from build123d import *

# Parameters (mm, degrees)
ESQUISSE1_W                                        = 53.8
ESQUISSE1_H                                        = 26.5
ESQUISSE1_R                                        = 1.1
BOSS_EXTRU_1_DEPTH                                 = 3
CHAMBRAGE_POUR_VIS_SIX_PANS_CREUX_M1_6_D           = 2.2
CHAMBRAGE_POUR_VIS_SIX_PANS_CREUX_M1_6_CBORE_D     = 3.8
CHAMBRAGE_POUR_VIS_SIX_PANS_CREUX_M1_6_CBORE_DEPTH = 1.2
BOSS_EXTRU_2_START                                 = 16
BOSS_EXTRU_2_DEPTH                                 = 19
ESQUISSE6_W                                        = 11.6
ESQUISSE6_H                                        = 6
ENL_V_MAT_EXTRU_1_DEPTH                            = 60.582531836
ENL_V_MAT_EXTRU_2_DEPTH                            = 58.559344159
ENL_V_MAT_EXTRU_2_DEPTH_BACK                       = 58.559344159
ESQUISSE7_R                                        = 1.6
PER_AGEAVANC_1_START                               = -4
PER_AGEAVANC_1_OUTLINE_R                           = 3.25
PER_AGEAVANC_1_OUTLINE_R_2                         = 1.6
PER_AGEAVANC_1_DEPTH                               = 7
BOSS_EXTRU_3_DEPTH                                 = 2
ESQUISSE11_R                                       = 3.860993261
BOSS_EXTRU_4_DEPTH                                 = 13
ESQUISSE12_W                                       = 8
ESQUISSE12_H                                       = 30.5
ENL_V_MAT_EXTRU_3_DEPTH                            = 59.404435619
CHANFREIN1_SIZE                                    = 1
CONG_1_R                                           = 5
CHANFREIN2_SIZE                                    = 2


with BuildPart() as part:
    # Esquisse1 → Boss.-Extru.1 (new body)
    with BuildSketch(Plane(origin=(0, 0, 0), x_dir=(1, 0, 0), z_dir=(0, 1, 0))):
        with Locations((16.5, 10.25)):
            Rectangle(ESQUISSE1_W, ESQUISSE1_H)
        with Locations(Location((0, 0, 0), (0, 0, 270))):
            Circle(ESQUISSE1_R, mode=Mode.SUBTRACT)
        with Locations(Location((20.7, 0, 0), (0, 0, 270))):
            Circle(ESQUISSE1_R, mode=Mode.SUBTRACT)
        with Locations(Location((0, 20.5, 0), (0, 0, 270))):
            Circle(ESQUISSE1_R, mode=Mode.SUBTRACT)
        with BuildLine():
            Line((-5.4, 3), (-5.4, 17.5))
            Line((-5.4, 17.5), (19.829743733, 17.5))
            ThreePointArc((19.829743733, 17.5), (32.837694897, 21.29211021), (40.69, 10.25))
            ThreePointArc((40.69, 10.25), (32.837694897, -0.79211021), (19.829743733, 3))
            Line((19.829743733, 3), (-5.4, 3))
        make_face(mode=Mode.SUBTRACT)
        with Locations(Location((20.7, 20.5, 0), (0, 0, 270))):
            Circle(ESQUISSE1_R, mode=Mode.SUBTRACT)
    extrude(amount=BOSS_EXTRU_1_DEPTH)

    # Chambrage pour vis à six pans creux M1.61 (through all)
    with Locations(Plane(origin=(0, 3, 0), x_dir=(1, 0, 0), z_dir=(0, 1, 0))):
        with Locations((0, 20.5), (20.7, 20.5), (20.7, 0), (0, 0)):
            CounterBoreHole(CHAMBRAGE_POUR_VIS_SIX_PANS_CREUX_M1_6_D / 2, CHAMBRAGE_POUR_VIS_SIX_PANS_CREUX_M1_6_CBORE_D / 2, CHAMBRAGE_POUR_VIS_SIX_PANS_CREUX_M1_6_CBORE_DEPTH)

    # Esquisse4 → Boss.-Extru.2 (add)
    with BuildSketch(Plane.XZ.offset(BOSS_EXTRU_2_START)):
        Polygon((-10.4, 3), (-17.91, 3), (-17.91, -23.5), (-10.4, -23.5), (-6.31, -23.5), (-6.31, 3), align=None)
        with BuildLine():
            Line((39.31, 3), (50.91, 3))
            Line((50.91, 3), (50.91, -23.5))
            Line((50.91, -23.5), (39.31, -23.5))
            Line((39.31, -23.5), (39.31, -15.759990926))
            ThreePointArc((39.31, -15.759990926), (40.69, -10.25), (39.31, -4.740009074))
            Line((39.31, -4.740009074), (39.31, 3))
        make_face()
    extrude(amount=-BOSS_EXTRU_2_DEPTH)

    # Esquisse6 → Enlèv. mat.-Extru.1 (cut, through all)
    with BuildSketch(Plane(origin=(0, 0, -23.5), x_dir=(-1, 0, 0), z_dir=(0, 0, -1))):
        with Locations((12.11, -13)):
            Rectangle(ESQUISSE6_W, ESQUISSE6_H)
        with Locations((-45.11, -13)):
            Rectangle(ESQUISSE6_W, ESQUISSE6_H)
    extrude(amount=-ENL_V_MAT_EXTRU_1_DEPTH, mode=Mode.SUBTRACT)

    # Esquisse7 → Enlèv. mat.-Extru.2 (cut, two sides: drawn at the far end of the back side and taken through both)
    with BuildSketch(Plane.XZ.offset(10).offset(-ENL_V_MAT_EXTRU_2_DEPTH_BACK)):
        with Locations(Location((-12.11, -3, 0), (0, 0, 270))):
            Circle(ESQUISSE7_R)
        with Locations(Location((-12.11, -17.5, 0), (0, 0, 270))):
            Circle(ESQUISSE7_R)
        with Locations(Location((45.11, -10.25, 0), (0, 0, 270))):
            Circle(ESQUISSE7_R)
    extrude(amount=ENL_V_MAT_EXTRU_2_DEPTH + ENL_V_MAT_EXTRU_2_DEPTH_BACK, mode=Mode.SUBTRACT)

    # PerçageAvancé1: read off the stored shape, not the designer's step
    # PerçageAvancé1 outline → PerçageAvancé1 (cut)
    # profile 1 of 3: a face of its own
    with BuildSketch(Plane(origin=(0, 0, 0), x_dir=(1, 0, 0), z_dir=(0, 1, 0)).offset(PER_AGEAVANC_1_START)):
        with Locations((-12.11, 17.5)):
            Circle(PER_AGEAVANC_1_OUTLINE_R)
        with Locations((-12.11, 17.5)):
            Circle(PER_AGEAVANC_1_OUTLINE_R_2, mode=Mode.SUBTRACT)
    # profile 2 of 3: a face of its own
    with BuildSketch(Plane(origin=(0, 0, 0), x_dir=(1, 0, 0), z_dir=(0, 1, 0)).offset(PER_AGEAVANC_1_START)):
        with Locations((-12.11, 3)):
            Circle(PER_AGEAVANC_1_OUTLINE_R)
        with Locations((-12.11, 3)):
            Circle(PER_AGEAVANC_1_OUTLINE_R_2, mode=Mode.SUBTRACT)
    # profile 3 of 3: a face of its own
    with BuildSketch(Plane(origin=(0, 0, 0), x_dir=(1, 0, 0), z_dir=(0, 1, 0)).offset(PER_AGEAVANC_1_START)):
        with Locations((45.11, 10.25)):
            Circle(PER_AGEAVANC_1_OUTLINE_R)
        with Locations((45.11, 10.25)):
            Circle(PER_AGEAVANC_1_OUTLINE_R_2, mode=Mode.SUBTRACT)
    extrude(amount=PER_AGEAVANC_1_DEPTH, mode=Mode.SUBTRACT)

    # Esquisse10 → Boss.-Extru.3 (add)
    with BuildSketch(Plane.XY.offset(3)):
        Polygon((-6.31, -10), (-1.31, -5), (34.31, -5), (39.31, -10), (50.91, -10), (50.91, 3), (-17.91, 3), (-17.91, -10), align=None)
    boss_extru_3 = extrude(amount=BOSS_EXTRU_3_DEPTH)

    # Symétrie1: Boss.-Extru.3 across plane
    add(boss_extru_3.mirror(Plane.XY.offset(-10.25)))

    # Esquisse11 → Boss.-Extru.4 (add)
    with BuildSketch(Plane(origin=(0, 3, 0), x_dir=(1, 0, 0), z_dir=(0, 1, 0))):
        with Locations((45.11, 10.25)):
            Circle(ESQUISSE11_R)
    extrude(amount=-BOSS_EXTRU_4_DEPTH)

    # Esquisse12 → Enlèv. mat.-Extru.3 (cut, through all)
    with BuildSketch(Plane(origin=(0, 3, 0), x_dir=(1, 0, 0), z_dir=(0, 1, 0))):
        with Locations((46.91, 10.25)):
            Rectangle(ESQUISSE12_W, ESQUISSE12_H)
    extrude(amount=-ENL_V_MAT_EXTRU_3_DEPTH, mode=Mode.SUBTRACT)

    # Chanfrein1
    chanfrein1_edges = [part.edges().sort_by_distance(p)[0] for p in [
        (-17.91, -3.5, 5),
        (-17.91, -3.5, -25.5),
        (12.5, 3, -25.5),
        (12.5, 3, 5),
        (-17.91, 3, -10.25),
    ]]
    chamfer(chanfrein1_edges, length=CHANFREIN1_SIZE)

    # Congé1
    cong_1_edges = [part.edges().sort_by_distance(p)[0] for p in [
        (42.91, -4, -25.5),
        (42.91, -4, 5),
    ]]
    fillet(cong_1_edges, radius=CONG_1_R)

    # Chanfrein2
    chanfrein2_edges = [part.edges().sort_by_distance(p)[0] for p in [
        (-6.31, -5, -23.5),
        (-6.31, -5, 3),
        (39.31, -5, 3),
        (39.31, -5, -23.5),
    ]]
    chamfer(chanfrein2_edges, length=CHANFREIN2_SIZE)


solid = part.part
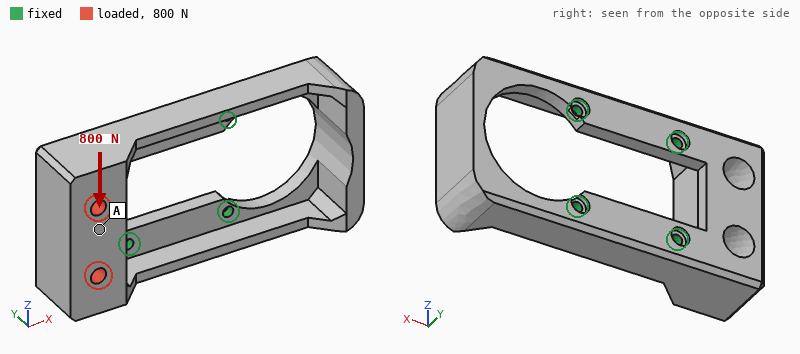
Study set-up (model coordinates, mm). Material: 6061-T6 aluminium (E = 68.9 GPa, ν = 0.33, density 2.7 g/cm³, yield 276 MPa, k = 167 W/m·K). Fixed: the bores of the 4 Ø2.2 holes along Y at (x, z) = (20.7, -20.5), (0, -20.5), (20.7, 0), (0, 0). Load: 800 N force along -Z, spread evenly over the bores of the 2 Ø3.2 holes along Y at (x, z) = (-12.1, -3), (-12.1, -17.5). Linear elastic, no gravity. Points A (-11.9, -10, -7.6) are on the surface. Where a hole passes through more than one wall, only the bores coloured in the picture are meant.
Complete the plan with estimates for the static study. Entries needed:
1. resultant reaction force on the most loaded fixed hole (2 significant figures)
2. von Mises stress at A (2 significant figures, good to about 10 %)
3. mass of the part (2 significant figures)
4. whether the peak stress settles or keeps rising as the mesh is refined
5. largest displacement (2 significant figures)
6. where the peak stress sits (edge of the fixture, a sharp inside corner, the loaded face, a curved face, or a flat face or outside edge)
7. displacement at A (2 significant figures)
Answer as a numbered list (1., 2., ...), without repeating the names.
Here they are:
1. 550 N
2. 14 MPa
3. 22 g
4. keeps rising
5. 28 µm
6. edge of the fixture
7. 23 µm
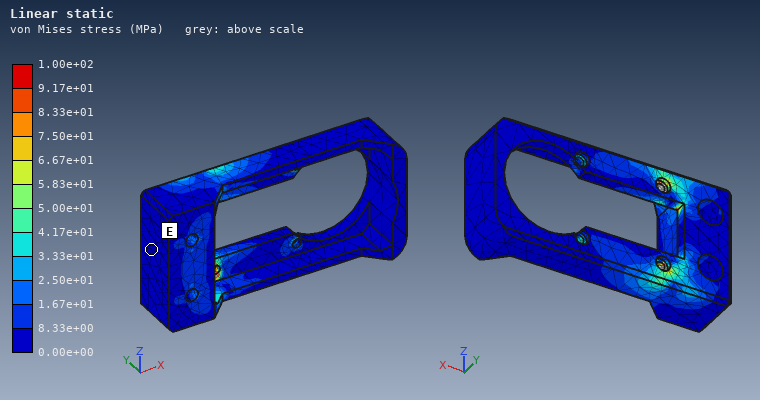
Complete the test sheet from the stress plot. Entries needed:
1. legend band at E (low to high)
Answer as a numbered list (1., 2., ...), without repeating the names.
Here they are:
1. 0.00e+00 to 8.33e+00 MPa
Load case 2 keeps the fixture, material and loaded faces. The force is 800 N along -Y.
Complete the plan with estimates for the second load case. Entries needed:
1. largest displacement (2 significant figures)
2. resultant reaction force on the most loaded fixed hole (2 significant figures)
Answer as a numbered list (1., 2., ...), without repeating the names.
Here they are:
1. 0.12 mm
2. 600 N
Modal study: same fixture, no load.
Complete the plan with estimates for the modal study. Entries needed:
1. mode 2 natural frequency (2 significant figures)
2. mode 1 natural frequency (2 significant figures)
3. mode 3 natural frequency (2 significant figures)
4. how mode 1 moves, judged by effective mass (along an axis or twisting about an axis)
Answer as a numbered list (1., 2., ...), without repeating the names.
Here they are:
1. 4600 Hz
2. 3800 Hz
3. 4600 Hz
4. along Y
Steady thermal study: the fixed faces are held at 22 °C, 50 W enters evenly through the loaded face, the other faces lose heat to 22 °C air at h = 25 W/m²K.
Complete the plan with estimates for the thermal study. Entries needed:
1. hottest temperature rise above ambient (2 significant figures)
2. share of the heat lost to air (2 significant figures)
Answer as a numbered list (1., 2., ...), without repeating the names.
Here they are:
1. 55 K
2. 5.5 %
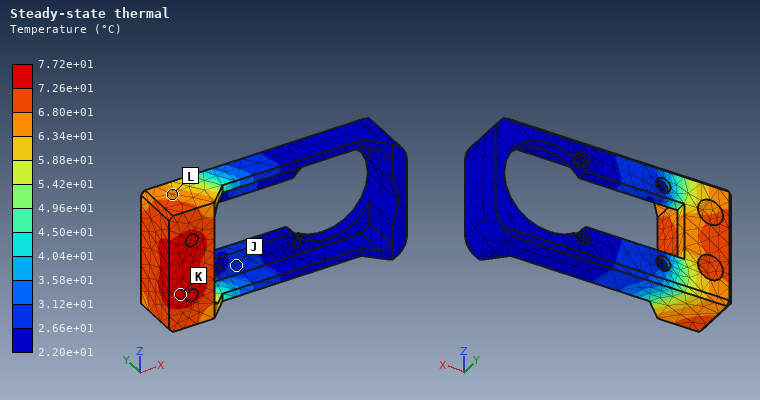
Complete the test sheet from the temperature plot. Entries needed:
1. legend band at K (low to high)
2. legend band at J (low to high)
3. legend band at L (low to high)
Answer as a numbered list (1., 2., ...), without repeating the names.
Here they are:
1. 7.26e+01 to 7.72e+01 °C
2. 2.66e+01 to 3.12e+01 °C
3. 6.34e+01 to 6.80e+01 °C
